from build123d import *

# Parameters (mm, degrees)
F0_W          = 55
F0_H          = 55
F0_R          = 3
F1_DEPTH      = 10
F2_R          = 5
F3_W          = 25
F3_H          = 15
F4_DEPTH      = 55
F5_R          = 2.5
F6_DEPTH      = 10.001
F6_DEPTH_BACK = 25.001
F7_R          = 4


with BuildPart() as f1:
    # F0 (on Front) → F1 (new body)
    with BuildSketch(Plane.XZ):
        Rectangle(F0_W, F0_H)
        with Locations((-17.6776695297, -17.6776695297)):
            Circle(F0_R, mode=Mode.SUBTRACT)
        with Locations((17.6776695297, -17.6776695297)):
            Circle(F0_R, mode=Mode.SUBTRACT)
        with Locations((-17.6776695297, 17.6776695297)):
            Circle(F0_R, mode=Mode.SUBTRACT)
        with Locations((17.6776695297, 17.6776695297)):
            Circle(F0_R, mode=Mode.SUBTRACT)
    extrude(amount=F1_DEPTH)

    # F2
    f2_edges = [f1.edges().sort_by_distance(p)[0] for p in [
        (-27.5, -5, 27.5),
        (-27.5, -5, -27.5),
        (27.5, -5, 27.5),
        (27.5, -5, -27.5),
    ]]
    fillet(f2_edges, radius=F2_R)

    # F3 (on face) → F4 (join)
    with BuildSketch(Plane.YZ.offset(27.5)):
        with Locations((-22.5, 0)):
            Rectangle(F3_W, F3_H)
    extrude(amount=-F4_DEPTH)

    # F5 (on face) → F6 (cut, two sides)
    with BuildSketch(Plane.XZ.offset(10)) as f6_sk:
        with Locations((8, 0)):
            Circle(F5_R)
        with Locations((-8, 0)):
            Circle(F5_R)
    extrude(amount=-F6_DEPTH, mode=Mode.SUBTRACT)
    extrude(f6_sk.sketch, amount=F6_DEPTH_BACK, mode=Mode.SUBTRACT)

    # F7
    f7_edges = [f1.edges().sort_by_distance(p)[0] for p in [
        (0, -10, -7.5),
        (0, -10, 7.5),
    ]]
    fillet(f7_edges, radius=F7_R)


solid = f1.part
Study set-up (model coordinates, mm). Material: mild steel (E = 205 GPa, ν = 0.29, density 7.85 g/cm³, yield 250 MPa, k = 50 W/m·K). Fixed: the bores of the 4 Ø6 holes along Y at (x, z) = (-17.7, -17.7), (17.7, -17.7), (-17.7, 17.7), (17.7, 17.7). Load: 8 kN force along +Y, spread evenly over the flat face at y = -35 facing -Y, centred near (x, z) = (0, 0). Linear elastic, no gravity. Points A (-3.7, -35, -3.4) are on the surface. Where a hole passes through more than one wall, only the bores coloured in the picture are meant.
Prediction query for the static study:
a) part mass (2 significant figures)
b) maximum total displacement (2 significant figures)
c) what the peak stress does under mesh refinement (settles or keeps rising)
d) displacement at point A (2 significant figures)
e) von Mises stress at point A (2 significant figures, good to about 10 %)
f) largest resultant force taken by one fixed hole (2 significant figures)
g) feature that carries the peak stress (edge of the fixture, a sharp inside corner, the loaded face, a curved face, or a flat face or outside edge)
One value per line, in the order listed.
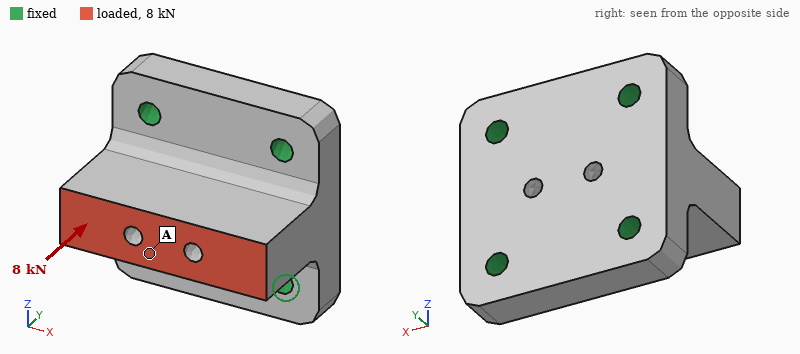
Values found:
380 g
3.5 µm
keeps rising
3.5 µm
9.8 MPa
2.1 kN
edge of the fixture
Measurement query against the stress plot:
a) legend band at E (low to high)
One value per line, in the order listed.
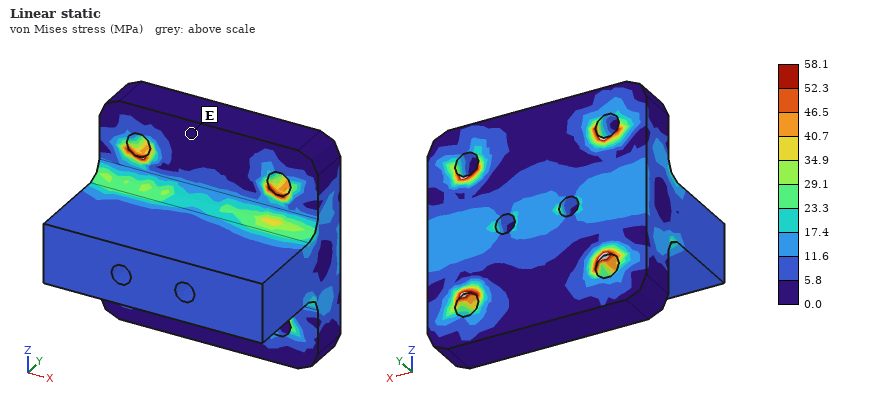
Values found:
0.0 to 5.8 MPa
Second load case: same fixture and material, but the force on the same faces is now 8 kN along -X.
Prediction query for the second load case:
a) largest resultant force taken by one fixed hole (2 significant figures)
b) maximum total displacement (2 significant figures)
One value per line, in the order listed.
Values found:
3.8 kN
16 µm
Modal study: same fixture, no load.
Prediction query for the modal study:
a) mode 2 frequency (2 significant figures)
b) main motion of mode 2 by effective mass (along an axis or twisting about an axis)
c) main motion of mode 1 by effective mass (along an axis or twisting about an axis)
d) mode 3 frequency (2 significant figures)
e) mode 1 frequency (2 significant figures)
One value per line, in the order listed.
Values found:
13 kHz
along X
along Z
18 kHz
12 kHz
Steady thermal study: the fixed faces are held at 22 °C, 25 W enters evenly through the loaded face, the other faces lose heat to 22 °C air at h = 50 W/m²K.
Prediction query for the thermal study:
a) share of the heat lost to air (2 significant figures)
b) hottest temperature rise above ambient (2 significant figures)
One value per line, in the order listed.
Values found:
15 %
21 K
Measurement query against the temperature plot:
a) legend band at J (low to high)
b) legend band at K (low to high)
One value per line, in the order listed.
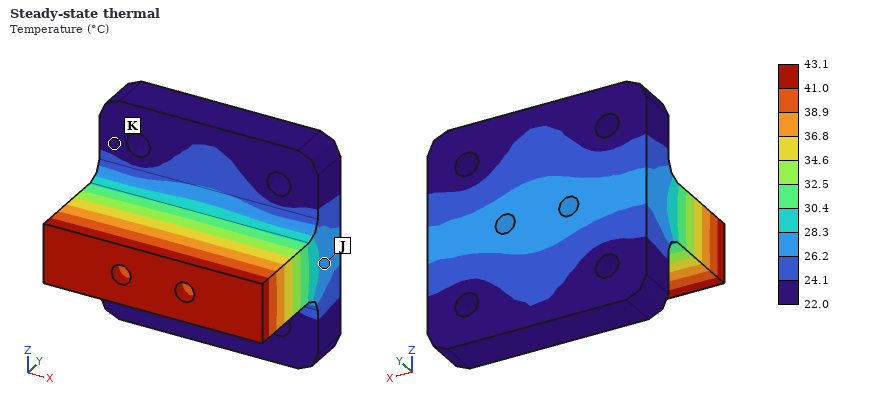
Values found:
26.2 to 28.3 °C
22.0 to 24.1 °C
